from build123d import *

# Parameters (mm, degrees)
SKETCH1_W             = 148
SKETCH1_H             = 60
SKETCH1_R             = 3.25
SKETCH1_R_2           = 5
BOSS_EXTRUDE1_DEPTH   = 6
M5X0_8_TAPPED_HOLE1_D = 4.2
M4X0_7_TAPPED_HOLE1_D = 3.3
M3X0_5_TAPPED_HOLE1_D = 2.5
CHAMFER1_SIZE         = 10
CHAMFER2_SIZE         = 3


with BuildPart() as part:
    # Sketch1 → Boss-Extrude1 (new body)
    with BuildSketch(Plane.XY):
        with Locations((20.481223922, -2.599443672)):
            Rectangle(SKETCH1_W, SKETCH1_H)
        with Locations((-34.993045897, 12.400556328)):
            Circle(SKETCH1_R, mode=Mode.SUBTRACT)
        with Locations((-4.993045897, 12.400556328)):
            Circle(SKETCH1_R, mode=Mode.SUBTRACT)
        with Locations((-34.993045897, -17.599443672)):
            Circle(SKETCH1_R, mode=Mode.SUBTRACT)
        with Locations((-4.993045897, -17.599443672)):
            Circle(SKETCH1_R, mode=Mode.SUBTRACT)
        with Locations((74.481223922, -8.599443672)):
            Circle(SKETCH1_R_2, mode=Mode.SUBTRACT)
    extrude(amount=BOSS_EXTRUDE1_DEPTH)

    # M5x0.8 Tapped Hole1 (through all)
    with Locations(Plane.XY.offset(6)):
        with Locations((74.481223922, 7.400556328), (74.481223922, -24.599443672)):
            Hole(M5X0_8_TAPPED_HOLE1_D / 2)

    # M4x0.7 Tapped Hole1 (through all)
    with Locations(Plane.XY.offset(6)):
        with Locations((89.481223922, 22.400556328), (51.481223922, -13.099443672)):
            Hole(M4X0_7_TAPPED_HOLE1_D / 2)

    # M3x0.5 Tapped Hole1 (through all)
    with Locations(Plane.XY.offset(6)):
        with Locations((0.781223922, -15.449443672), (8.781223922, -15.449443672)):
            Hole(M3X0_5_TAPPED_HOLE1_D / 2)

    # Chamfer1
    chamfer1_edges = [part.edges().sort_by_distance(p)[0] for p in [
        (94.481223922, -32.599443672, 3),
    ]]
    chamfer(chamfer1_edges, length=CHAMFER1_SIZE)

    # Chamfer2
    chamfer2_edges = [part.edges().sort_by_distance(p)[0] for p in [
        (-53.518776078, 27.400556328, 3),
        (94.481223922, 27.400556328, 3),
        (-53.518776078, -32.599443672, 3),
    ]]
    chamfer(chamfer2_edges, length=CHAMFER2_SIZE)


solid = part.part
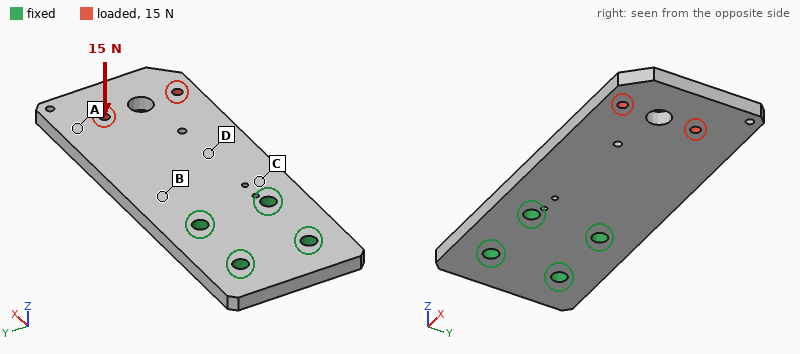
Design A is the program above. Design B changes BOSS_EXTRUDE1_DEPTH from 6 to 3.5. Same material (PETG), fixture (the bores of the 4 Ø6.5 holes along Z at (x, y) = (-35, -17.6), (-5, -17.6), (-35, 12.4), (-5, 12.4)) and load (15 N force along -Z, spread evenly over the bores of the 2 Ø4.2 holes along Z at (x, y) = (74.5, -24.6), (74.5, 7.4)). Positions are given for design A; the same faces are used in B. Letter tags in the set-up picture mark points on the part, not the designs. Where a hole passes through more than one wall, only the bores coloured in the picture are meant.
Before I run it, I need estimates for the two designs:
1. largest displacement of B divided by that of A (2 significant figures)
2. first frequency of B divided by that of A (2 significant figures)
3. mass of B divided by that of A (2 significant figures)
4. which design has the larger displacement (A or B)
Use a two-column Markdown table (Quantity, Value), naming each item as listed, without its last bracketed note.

| Quantity | Value |
|---|---|
| largest displacement of B divided by that of A | 4.9 |
| first frequency of B divided by that of A | 0.59 |
| mass of B divided by that of A | 0.58 |
| which design has the larger displacement | B |
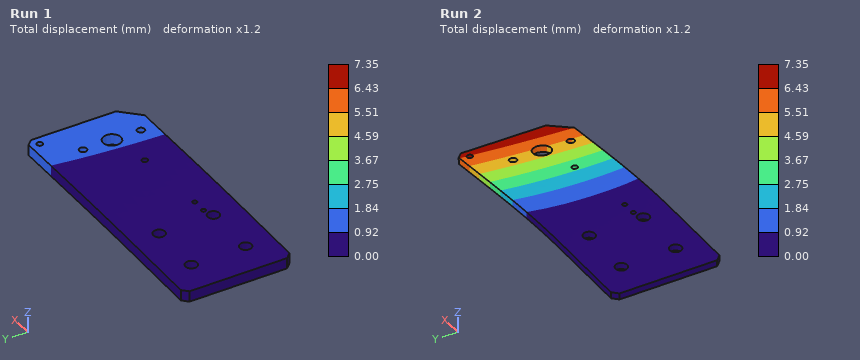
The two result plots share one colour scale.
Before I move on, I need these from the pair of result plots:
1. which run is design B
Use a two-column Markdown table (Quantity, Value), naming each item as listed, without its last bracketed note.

| Quantity | Value |
|---|---|
| which run is design B | Run 2 |
